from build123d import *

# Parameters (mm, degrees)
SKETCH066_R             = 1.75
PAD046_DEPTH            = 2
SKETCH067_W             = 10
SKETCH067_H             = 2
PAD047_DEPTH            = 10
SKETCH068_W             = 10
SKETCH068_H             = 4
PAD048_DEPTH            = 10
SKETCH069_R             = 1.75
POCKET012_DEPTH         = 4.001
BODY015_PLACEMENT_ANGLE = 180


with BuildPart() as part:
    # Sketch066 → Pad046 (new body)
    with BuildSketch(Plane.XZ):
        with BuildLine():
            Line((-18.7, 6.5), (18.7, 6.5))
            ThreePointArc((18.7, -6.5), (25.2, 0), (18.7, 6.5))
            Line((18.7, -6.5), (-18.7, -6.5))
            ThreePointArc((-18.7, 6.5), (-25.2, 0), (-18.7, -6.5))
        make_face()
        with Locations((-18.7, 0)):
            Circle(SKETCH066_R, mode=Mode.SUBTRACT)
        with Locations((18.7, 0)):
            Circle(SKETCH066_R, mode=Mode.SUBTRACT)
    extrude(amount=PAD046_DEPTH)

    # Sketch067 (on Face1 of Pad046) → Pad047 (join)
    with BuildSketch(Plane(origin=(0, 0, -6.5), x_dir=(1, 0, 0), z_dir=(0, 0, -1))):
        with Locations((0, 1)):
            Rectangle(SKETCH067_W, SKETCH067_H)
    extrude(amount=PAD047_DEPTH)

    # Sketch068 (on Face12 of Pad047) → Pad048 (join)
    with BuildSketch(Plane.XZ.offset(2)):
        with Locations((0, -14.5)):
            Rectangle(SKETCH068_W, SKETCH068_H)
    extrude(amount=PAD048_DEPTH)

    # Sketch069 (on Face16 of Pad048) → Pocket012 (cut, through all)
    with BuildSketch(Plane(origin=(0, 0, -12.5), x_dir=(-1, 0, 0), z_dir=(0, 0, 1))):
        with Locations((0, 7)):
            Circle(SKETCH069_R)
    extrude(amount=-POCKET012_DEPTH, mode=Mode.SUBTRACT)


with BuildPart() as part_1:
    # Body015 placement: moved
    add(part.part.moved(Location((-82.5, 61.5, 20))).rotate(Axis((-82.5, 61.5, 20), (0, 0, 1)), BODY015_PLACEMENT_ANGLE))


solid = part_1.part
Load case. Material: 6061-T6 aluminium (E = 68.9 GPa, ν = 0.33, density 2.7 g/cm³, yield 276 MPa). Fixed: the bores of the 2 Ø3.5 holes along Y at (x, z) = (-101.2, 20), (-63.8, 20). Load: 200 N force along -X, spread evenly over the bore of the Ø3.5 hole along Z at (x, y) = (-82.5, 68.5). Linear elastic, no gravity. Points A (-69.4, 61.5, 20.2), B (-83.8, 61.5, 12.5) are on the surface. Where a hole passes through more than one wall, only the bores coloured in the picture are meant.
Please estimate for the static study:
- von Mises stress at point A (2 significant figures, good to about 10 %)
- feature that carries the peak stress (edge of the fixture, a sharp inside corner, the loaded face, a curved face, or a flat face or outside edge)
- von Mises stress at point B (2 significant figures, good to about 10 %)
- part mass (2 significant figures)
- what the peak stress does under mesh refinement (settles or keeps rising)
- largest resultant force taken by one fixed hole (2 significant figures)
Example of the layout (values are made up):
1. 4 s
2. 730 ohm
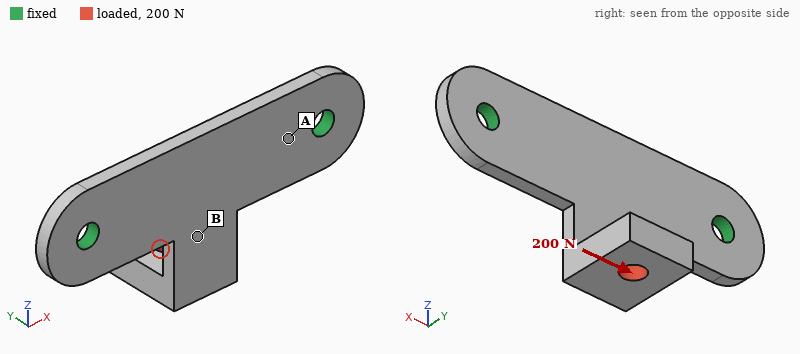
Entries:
1. 30 MPa
2. a sharp inside corner
3. 110 MPa
4. 4.8 g
5. keeps rising
6. 140 N
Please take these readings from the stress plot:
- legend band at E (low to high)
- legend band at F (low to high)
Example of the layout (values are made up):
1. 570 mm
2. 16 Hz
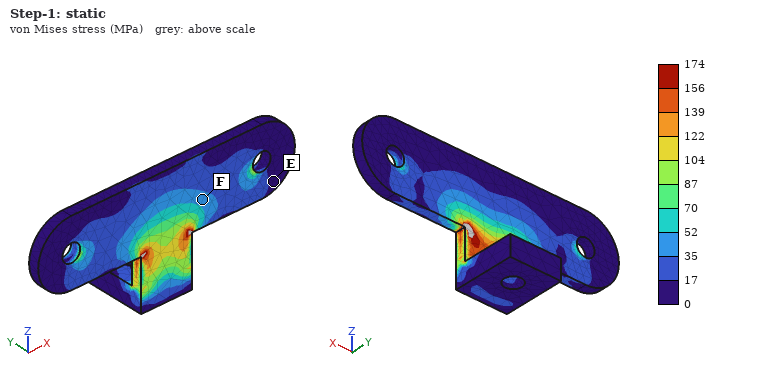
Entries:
1. 0 to 17 MPa
2. 35 to 52 MPa
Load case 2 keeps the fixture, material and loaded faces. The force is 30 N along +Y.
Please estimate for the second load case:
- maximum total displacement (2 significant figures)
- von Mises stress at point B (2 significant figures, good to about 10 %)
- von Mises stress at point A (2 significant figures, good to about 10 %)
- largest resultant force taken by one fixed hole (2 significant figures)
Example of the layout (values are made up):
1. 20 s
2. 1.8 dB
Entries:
1. 0.13 mm
2. 32 MPa
3. 23 MPa
4. 15 N
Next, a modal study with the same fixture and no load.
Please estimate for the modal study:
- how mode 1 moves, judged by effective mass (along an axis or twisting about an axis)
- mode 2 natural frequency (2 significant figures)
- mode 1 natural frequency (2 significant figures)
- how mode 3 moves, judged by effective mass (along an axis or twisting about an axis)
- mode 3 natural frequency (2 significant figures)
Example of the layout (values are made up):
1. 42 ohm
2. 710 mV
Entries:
1. along Y
2. 5600 Hz
3. 2200 Hz
4. along Y
5. 6600 Hz
